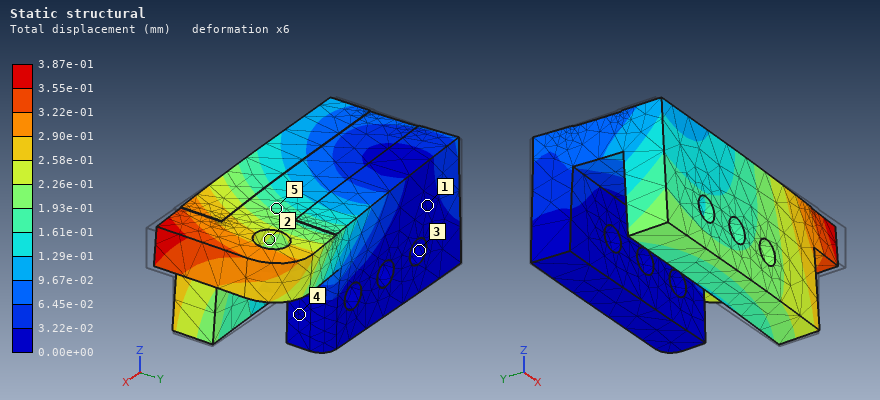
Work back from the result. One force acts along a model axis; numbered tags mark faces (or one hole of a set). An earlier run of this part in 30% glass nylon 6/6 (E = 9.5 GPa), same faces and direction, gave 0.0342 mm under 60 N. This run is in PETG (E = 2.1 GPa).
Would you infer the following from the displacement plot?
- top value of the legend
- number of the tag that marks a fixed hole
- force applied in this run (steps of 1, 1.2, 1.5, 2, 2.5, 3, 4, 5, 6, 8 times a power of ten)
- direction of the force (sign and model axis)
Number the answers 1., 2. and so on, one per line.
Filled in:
1. 3.87e-01 mm
2. 3
3. 150 N
4. +Y
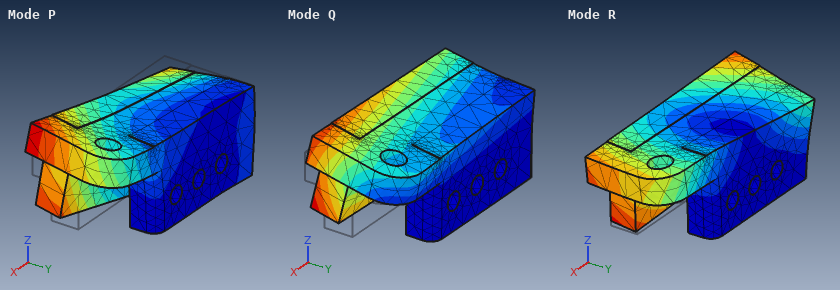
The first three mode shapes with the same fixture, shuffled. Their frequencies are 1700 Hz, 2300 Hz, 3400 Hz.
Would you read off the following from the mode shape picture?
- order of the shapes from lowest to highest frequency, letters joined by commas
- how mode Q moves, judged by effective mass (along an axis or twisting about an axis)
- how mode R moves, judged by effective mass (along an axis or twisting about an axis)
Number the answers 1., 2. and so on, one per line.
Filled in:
1. Q, R, P
2. along Z
3. along X
